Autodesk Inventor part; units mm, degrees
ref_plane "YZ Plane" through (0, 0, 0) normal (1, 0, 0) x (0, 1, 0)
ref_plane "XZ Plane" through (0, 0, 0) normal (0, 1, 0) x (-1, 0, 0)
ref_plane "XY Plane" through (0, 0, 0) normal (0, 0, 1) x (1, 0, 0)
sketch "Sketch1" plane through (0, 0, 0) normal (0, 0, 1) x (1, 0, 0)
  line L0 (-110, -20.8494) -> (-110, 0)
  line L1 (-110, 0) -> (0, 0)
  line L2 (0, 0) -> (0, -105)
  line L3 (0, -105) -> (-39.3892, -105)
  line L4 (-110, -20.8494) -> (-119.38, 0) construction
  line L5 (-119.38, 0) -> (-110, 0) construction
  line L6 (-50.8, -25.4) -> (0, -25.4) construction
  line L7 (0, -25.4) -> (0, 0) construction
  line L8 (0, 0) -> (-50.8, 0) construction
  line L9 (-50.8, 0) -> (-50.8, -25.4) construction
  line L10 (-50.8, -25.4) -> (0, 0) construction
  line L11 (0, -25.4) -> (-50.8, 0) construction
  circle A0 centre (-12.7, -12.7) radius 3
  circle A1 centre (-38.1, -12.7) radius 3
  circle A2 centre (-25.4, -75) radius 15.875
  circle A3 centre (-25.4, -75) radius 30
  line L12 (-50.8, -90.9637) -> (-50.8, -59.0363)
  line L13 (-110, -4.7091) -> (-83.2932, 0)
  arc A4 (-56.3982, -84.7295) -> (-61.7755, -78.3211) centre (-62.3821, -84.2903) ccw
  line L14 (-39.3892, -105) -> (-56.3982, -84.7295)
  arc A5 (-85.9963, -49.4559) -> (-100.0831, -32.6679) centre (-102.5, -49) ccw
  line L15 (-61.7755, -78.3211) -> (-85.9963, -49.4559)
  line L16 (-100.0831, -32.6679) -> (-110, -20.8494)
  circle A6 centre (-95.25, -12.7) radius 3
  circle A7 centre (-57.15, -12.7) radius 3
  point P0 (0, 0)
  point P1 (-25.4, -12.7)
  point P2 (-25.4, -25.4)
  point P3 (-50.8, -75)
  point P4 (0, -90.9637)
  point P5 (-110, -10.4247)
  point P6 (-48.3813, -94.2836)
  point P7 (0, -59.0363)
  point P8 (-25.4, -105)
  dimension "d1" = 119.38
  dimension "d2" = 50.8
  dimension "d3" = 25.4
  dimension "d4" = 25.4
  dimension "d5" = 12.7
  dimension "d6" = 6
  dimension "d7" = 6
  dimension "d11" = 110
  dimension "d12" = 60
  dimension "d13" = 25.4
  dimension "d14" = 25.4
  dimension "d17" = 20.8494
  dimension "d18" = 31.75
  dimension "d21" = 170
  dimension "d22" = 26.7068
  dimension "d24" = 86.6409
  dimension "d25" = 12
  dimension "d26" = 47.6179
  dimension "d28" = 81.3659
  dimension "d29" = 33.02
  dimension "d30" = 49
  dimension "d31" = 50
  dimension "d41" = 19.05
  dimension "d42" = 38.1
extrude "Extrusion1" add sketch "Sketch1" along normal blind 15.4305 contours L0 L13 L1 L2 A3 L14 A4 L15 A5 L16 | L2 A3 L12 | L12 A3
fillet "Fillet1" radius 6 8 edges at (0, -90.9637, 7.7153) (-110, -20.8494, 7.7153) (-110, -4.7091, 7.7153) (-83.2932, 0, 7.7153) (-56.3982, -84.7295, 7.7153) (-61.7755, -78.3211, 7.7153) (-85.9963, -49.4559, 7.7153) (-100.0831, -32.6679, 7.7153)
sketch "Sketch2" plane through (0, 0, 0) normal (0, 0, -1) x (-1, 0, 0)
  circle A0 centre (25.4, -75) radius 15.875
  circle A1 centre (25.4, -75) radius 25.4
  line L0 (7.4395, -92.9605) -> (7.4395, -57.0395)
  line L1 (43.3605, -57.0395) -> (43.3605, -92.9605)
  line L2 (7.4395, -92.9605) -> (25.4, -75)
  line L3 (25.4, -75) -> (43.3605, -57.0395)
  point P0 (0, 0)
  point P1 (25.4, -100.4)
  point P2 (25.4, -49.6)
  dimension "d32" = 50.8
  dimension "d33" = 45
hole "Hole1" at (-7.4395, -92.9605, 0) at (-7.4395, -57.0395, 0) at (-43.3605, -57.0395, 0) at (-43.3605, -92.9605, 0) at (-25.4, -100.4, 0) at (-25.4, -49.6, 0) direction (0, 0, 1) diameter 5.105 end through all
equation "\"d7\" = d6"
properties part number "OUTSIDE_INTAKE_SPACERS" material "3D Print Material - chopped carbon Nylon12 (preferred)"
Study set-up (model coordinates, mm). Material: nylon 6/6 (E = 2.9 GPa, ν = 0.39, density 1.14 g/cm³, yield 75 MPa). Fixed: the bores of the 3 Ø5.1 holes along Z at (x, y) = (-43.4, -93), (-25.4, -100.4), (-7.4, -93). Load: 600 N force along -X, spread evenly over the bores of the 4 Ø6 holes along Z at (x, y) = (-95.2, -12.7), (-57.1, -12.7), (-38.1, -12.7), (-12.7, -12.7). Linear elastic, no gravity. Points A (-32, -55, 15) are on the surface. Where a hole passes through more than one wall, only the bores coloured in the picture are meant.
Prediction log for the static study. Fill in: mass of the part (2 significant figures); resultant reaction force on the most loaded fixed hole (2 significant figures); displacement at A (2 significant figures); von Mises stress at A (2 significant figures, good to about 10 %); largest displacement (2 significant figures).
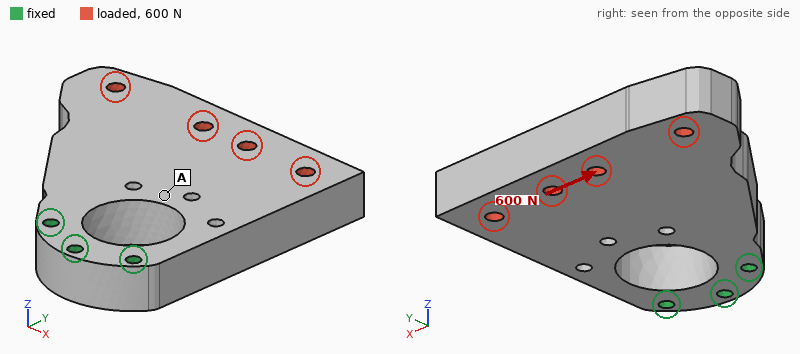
130 g
1.2 kN
0.28 mm
2.8 MPa
0.71 mm
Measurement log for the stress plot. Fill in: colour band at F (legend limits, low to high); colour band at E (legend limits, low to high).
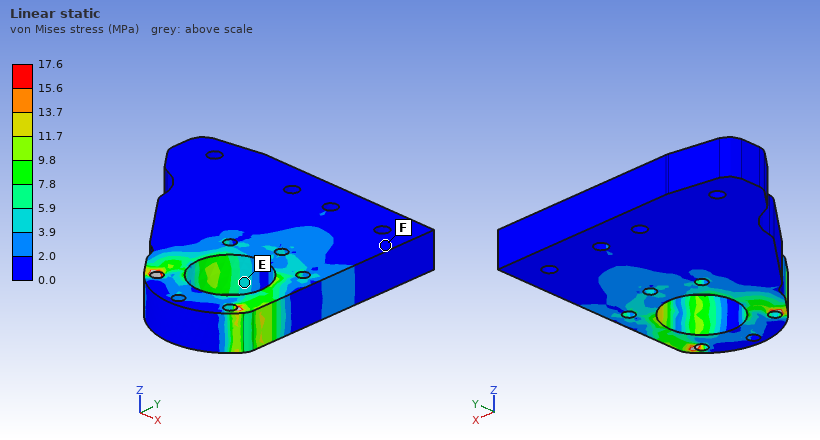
0.0 to 2.0 MPa
3.9 to 5.9 MPa
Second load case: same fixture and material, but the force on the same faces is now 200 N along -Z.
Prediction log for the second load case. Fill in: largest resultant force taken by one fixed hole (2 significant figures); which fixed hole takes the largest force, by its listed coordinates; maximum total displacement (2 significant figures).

210 N
(-43.4, -93)
1.8 mm
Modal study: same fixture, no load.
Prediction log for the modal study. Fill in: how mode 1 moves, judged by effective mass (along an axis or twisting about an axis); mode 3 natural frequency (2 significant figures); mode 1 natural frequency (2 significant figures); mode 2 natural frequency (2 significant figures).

along Z
580 Hz
240 Hz
570 Hz
